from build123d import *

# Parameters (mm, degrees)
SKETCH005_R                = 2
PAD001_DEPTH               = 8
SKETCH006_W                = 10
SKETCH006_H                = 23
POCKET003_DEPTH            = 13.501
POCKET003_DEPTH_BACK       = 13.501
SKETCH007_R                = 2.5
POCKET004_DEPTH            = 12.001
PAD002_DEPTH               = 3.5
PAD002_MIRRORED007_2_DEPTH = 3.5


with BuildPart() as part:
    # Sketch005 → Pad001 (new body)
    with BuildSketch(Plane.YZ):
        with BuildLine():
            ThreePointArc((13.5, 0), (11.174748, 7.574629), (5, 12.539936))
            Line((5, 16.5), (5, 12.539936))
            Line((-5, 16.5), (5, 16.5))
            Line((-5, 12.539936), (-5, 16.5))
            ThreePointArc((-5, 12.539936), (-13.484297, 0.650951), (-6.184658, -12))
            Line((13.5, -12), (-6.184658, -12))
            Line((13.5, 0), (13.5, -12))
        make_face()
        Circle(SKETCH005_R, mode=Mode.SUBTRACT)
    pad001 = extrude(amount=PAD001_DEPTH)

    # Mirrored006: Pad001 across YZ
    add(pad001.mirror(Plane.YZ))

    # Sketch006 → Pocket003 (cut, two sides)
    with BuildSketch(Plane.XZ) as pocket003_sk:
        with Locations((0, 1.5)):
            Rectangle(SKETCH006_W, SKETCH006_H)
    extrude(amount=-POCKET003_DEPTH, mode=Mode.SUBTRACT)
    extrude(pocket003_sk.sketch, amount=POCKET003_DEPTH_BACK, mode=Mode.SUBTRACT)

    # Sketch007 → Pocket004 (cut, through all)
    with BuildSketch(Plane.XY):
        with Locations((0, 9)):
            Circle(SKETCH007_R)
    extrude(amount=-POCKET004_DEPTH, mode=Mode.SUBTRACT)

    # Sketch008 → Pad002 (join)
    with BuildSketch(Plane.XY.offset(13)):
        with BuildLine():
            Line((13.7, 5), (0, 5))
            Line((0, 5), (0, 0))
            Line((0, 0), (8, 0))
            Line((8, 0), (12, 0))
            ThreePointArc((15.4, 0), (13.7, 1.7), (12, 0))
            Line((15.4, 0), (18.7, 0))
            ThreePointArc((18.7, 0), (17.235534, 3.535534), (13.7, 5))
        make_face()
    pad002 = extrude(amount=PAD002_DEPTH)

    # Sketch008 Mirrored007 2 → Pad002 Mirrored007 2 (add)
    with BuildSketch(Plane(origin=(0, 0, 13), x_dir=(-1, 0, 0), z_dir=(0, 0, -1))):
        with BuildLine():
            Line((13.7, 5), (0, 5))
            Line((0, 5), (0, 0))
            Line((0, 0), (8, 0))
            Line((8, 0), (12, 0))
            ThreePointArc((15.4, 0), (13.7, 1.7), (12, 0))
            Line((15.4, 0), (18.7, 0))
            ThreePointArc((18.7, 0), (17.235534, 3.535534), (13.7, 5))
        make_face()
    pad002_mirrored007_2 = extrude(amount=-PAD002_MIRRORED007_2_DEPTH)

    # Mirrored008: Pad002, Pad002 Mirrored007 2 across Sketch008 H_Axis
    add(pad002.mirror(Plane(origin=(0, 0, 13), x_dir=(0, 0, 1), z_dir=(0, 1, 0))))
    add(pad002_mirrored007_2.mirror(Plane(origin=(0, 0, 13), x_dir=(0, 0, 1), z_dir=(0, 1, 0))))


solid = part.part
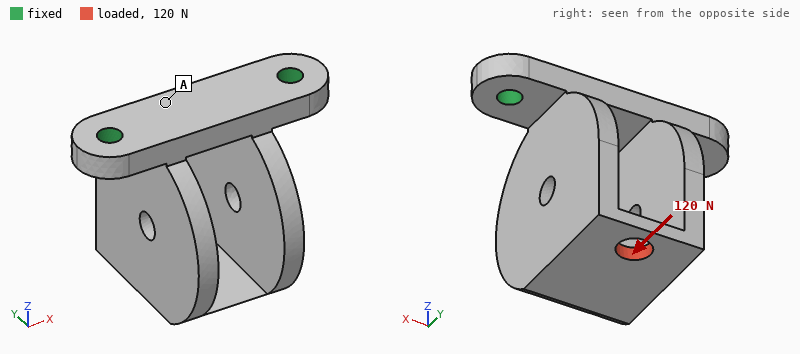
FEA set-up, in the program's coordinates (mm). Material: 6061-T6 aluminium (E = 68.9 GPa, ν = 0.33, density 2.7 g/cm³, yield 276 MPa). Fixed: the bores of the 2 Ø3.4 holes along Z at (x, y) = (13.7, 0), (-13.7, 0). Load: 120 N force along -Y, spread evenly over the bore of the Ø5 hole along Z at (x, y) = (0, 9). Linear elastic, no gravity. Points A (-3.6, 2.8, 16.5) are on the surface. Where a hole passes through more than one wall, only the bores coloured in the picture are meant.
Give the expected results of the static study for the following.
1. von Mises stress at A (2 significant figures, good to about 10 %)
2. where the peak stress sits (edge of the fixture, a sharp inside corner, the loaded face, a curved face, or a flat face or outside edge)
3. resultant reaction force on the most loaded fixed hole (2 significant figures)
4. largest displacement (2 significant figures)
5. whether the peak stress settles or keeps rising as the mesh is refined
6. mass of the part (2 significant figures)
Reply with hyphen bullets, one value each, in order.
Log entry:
- 11 MPa
- edge of the fixture
- 60 N
- 87 µm
- keeps rising
- 13 g
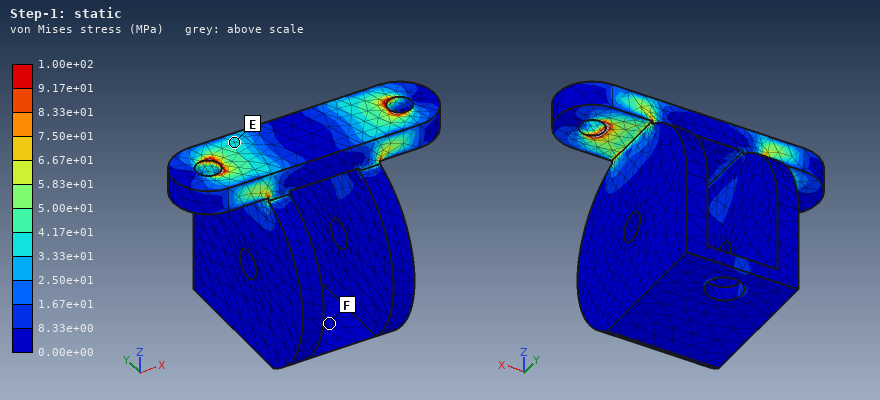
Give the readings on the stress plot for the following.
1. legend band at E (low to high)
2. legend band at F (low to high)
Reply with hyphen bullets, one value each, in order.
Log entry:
- 3.33e+01 to 4.17e+01 MPa
- 0.00e+00 to 8.33e+00 MPa
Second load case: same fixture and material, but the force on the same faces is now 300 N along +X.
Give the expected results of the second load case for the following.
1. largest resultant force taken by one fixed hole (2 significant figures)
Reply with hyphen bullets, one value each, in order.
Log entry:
- 400 N
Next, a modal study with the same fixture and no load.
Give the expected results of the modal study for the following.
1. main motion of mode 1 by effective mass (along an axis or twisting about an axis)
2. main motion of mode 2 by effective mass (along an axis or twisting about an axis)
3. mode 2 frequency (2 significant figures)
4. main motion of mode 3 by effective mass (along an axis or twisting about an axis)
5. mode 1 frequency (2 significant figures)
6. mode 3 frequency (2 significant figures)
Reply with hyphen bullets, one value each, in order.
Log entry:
- along Y
- along X
- 3500 Hz
- twisting about Z
- 2700 Hz
- 5600 Hz
